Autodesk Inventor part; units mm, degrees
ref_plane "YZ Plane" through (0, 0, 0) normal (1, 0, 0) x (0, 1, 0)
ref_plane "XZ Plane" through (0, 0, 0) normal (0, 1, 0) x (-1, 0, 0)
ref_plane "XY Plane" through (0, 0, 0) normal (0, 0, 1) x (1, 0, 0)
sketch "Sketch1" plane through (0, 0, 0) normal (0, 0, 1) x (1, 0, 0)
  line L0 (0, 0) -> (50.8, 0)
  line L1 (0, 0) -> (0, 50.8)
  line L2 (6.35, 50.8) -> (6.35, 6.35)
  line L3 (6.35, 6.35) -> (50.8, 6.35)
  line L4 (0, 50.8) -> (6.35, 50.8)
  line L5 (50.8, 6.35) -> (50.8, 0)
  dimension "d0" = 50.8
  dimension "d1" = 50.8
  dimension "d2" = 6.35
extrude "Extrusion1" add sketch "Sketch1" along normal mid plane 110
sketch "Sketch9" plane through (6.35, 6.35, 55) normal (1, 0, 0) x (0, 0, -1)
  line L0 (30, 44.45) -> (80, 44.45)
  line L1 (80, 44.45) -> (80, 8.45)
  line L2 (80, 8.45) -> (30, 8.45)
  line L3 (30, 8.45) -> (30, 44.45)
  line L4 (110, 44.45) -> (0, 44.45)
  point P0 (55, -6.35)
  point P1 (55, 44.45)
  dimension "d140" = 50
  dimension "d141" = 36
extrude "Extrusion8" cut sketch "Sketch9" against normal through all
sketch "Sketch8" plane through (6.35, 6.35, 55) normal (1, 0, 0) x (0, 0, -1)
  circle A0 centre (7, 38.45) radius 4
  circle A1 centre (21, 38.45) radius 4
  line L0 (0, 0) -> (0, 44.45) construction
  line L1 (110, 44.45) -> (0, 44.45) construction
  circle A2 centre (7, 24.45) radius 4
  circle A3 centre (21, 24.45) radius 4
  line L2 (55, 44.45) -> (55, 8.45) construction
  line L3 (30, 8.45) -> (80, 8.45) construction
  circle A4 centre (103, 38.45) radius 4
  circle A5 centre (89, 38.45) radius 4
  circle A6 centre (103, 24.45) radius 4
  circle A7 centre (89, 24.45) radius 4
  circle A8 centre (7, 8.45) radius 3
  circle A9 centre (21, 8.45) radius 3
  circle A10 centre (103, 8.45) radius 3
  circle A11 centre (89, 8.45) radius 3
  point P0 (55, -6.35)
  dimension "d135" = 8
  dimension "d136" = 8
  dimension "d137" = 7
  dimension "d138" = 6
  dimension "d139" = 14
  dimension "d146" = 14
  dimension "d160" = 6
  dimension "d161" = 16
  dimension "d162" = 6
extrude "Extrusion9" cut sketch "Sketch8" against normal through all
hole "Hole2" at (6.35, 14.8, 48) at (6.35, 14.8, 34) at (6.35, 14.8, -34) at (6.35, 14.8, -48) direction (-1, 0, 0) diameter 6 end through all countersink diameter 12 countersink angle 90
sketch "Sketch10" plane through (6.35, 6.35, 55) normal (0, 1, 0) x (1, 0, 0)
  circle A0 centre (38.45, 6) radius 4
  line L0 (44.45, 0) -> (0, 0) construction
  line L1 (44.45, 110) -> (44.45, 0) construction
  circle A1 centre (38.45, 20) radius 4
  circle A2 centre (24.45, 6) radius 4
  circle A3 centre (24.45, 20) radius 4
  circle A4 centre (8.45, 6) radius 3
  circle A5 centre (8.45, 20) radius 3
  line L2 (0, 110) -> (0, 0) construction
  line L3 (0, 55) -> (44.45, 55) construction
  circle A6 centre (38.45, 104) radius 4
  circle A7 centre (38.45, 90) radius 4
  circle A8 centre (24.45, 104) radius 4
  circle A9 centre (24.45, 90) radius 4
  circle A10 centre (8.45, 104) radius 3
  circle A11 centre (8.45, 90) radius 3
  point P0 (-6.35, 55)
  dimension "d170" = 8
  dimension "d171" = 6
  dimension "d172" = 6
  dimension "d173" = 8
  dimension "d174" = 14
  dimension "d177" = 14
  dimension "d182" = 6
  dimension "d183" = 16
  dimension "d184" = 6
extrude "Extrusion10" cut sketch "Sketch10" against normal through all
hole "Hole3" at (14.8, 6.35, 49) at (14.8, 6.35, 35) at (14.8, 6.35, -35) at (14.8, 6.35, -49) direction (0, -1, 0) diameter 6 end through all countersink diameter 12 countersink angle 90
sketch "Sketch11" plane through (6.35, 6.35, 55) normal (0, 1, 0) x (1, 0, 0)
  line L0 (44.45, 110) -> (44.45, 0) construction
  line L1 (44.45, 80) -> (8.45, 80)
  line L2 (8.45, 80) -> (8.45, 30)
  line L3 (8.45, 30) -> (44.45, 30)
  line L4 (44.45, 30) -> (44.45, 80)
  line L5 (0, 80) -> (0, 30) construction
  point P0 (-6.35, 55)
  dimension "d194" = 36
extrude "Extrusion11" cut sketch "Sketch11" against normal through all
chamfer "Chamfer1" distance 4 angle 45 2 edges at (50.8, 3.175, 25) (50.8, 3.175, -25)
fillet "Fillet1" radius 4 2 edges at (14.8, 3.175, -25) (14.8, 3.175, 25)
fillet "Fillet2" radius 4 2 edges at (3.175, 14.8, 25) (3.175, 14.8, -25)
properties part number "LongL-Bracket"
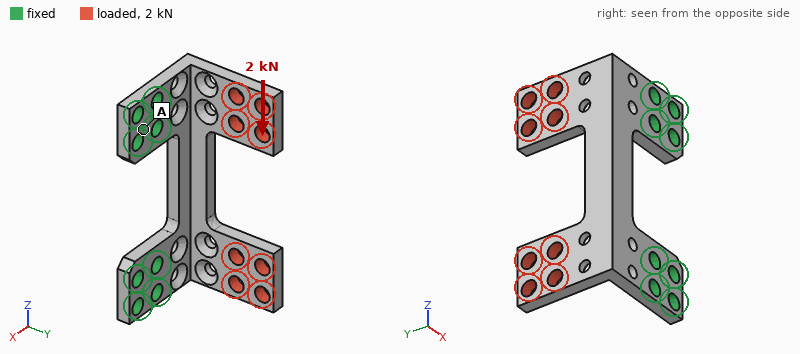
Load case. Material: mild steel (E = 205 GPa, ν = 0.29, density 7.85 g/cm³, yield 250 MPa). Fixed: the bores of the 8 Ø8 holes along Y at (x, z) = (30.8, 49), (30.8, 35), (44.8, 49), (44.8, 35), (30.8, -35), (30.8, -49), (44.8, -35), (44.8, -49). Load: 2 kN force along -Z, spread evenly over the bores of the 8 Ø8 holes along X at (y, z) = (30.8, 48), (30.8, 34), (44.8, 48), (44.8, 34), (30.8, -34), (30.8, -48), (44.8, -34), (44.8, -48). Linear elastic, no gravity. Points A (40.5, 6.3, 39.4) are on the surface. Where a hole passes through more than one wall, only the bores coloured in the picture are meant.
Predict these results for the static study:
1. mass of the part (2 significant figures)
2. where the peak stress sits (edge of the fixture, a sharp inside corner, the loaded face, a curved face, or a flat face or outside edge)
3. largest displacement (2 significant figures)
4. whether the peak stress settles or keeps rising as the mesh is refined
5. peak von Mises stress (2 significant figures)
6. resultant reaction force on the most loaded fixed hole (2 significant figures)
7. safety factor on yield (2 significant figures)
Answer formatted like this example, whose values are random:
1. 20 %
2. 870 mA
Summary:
1. 280 g
2. a curved face
3. 91 µm
4. settles
5. 150 MPa
6. 950 N
7. 1.7
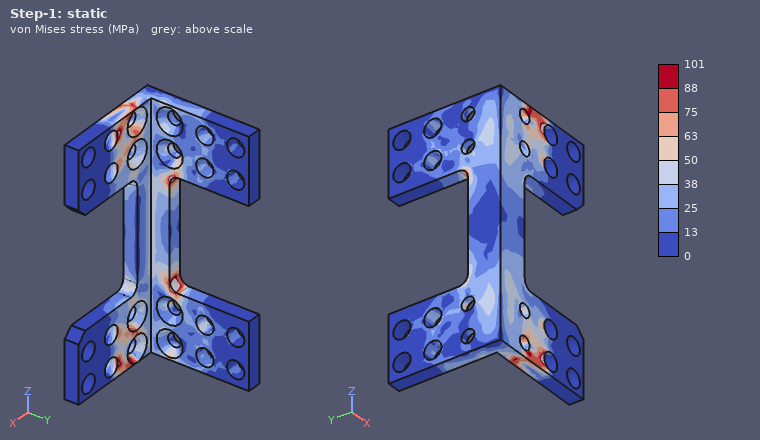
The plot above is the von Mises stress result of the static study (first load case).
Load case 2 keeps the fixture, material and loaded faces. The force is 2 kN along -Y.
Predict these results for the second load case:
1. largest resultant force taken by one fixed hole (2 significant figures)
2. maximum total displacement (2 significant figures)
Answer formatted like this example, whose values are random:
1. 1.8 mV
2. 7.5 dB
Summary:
1. 650 N
2. 0.16 mm
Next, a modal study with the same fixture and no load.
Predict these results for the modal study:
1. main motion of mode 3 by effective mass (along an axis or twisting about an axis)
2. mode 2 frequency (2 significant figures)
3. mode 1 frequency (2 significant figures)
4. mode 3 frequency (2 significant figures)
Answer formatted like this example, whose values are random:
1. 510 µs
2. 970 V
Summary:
1. along Y
2. 1600 Hz
3. 1200 Hz
4. 3300 Hz
